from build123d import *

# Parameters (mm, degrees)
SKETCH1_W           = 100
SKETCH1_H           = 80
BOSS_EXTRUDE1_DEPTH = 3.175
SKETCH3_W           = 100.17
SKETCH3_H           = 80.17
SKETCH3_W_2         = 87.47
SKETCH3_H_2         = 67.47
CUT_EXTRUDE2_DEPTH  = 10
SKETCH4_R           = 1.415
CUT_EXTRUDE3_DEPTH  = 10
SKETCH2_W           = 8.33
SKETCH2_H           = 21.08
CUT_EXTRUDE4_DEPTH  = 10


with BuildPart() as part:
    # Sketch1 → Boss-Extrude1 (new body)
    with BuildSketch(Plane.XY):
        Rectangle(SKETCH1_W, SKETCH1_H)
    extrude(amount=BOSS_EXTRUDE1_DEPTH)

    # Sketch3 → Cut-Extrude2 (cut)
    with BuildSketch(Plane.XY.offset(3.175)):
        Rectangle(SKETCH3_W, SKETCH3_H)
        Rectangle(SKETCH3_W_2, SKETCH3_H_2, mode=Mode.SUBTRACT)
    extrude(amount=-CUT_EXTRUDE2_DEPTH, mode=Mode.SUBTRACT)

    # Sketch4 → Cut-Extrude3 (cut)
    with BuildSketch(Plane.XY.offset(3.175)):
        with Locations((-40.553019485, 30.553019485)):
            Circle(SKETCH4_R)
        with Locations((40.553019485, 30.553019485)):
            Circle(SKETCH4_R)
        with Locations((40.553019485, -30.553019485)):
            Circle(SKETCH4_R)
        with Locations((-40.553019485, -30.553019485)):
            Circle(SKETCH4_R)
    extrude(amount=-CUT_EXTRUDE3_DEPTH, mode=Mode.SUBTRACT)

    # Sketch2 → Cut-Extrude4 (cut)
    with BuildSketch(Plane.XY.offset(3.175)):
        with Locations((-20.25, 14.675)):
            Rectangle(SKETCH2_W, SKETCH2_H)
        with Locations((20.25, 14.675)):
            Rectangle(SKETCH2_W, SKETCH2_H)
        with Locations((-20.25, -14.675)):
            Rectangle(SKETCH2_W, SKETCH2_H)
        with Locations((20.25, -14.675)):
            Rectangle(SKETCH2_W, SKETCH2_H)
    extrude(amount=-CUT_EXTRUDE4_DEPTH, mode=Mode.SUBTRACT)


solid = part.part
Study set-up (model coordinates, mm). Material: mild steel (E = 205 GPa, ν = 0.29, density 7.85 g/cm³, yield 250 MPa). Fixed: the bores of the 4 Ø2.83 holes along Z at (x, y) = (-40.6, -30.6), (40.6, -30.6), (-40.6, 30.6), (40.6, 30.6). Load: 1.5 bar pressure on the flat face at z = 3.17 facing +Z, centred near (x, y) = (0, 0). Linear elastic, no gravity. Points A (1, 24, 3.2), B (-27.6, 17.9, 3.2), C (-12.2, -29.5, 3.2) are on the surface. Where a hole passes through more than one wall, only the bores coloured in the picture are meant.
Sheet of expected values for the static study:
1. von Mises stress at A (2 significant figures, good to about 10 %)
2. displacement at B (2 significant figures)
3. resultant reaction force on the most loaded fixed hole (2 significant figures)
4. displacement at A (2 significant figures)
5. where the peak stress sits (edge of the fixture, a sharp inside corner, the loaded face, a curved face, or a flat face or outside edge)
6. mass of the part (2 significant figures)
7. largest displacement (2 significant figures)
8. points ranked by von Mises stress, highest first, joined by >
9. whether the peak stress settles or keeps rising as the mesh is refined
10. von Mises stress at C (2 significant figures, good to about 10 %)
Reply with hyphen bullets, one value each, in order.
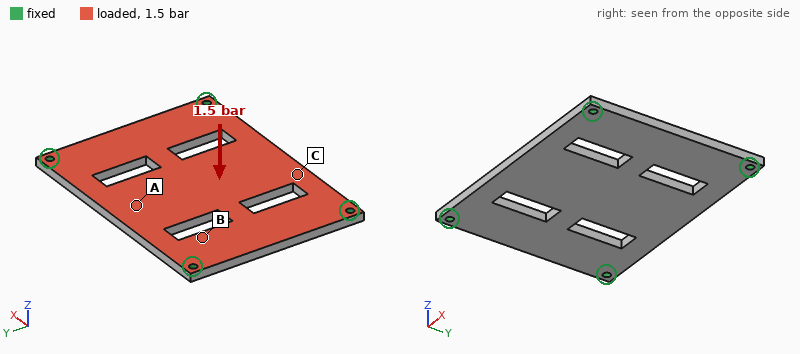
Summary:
- 26 MPa
- 30 µm
- 190 N
- 57 µm
- edge of the fixture
- 130 g
- 67 µm
- C > A > B
- keeps rising
- 36 MPa
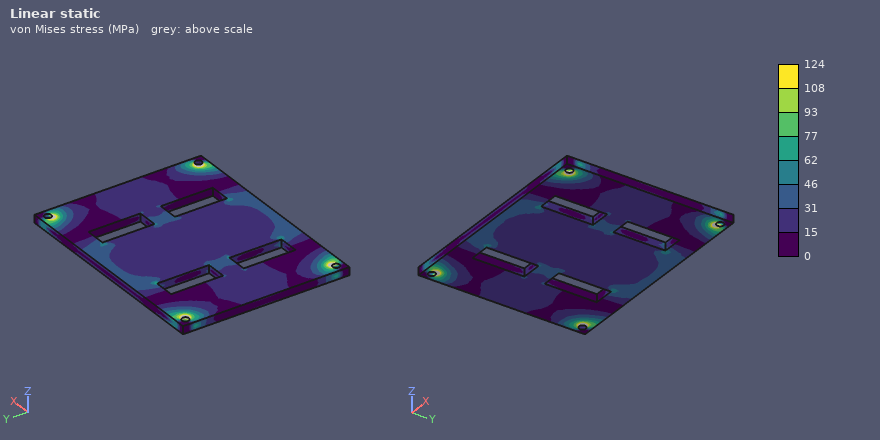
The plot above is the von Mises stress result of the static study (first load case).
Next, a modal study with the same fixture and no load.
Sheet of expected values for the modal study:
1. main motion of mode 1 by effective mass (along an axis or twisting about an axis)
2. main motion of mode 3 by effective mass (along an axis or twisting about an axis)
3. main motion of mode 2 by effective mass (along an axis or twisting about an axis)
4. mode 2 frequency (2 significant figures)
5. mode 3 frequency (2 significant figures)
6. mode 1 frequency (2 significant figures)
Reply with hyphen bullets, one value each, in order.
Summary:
- along Z
- twisting about Y
- twisting about X
- 2900 Hz
- 3800 Hz
- 1700 Hz
